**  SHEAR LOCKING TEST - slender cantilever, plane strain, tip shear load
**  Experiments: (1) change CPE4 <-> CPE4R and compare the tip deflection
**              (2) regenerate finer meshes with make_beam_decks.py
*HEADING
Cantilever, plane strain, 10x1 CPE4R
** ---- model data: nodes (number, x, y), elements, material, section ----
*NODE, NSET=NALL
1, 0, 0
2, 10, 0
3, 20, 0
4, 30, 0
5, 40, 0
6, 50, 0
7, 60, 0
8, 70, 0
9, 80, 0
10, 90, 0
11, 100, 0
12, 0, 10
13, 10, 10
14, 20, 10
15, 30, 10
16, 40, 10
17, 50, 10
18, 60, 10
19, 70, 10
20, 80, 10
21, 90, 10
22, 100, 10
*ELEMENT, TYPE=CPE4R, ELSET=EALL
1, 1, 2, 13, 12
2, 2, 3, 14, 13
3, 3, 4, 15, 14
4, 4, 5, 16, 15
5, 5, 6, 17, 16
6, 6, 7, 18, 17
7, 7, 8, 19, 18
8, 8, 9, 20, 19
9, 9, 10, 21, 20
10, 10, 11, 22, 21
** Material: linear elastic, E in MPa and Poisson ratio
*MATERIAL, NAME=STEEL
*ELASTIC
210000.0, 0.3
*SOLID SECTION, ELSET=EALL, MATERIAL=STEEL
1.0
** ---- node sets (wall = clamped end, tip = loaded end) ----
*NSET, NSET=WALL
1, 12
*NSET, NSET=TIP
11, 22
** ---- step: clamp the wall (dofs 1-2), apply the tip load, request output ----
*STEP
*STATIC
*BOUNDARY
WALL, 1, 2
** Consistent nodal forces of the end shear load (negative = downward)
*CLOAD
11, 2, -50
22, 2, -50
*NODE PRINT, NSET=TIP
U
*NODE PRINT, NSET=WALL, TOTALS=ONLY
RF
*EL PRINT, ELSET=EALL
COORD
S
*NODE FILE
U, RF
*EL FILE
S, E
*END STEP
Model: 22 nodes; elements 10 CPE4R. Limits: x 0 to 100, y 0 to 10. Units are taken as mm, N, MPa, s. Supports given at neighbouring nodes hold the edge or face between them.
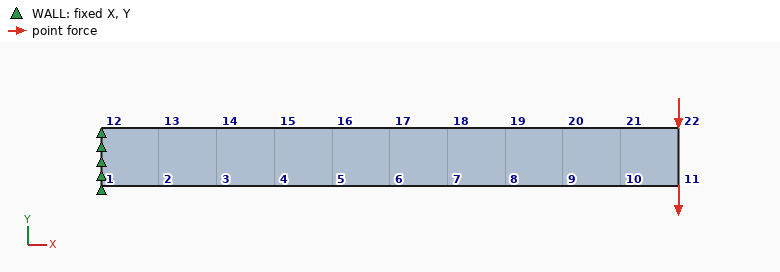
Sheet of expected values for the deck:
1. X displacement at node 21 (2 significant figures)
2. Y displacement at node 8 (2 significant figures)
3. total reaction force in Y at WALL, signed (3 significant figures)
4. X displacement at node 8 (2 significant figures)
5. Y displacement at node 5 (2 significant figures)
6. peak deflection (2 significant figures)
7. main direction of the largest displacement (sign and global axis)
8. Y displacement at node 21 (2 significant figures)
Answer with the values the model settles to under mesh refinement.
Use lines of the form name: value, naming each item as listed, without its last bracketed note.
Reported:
X displacement at node 21: 0.13 mm
Y displacement at node 8: -0.98 mm
total reaction force in Y at WALL, signed: 100 N
X displacement at node 8: -0.12 mm
Y displacement at node 5: -0.36 mm
peak deflection: 1.7 mm
main direction of the largest displacement: -Y
Y displacement at node 21: -1.5 mm
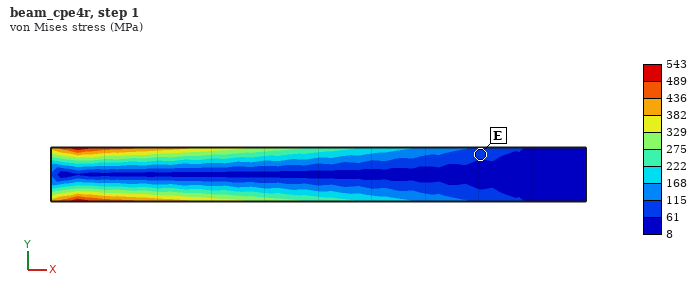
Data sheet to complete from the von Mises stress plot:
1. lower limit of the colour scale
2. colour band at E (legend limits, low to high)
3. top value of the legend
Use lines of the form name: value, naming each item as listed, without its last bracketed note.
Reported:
lower limit of the colour scale: 8 MPa
colour band at E: 61 to 115 MPa
top value of the legend: 543 MPa
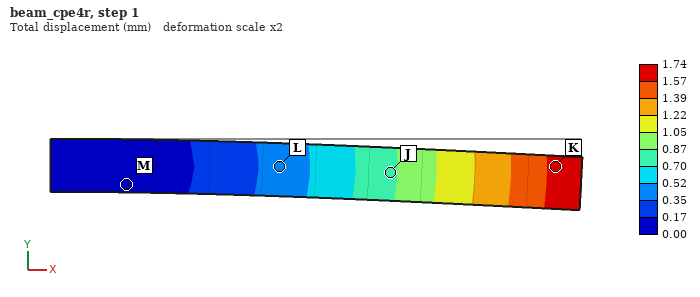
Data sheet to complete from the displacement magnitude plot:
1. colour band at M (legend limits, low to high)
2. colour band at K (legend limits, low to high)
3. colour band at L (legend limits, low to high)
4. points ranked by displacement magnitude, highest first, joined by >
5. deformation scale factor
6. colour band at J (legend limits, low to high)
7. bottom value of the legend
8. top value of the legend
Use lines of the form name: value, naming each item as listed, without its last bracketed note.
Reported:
colour band at M: 0.00 to 0.17 mm
colour band at K: 1.57 to 1.74 mm
colour band at L: 0.35 to 0.52 mm
points ranked by displacement magnitude, highest first, joined by >: K > J > L > M
deformation scale factor: 2
colour band at J: 0.70 to 0.87 mm
bottom value of the legend: 0.00 mm
top value of the legend: 1.74 mm
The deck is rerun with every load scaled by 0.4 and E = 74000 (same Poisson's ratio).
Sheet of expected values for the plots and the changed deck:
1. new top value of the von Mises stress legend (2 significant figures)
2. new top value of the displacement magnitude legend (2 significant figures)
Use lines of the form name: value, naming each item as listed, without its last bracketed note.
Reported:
new top value of the von Mises stress legend: 220 MPa
new top value of the displacement magnitude legend: 2.0 mm
